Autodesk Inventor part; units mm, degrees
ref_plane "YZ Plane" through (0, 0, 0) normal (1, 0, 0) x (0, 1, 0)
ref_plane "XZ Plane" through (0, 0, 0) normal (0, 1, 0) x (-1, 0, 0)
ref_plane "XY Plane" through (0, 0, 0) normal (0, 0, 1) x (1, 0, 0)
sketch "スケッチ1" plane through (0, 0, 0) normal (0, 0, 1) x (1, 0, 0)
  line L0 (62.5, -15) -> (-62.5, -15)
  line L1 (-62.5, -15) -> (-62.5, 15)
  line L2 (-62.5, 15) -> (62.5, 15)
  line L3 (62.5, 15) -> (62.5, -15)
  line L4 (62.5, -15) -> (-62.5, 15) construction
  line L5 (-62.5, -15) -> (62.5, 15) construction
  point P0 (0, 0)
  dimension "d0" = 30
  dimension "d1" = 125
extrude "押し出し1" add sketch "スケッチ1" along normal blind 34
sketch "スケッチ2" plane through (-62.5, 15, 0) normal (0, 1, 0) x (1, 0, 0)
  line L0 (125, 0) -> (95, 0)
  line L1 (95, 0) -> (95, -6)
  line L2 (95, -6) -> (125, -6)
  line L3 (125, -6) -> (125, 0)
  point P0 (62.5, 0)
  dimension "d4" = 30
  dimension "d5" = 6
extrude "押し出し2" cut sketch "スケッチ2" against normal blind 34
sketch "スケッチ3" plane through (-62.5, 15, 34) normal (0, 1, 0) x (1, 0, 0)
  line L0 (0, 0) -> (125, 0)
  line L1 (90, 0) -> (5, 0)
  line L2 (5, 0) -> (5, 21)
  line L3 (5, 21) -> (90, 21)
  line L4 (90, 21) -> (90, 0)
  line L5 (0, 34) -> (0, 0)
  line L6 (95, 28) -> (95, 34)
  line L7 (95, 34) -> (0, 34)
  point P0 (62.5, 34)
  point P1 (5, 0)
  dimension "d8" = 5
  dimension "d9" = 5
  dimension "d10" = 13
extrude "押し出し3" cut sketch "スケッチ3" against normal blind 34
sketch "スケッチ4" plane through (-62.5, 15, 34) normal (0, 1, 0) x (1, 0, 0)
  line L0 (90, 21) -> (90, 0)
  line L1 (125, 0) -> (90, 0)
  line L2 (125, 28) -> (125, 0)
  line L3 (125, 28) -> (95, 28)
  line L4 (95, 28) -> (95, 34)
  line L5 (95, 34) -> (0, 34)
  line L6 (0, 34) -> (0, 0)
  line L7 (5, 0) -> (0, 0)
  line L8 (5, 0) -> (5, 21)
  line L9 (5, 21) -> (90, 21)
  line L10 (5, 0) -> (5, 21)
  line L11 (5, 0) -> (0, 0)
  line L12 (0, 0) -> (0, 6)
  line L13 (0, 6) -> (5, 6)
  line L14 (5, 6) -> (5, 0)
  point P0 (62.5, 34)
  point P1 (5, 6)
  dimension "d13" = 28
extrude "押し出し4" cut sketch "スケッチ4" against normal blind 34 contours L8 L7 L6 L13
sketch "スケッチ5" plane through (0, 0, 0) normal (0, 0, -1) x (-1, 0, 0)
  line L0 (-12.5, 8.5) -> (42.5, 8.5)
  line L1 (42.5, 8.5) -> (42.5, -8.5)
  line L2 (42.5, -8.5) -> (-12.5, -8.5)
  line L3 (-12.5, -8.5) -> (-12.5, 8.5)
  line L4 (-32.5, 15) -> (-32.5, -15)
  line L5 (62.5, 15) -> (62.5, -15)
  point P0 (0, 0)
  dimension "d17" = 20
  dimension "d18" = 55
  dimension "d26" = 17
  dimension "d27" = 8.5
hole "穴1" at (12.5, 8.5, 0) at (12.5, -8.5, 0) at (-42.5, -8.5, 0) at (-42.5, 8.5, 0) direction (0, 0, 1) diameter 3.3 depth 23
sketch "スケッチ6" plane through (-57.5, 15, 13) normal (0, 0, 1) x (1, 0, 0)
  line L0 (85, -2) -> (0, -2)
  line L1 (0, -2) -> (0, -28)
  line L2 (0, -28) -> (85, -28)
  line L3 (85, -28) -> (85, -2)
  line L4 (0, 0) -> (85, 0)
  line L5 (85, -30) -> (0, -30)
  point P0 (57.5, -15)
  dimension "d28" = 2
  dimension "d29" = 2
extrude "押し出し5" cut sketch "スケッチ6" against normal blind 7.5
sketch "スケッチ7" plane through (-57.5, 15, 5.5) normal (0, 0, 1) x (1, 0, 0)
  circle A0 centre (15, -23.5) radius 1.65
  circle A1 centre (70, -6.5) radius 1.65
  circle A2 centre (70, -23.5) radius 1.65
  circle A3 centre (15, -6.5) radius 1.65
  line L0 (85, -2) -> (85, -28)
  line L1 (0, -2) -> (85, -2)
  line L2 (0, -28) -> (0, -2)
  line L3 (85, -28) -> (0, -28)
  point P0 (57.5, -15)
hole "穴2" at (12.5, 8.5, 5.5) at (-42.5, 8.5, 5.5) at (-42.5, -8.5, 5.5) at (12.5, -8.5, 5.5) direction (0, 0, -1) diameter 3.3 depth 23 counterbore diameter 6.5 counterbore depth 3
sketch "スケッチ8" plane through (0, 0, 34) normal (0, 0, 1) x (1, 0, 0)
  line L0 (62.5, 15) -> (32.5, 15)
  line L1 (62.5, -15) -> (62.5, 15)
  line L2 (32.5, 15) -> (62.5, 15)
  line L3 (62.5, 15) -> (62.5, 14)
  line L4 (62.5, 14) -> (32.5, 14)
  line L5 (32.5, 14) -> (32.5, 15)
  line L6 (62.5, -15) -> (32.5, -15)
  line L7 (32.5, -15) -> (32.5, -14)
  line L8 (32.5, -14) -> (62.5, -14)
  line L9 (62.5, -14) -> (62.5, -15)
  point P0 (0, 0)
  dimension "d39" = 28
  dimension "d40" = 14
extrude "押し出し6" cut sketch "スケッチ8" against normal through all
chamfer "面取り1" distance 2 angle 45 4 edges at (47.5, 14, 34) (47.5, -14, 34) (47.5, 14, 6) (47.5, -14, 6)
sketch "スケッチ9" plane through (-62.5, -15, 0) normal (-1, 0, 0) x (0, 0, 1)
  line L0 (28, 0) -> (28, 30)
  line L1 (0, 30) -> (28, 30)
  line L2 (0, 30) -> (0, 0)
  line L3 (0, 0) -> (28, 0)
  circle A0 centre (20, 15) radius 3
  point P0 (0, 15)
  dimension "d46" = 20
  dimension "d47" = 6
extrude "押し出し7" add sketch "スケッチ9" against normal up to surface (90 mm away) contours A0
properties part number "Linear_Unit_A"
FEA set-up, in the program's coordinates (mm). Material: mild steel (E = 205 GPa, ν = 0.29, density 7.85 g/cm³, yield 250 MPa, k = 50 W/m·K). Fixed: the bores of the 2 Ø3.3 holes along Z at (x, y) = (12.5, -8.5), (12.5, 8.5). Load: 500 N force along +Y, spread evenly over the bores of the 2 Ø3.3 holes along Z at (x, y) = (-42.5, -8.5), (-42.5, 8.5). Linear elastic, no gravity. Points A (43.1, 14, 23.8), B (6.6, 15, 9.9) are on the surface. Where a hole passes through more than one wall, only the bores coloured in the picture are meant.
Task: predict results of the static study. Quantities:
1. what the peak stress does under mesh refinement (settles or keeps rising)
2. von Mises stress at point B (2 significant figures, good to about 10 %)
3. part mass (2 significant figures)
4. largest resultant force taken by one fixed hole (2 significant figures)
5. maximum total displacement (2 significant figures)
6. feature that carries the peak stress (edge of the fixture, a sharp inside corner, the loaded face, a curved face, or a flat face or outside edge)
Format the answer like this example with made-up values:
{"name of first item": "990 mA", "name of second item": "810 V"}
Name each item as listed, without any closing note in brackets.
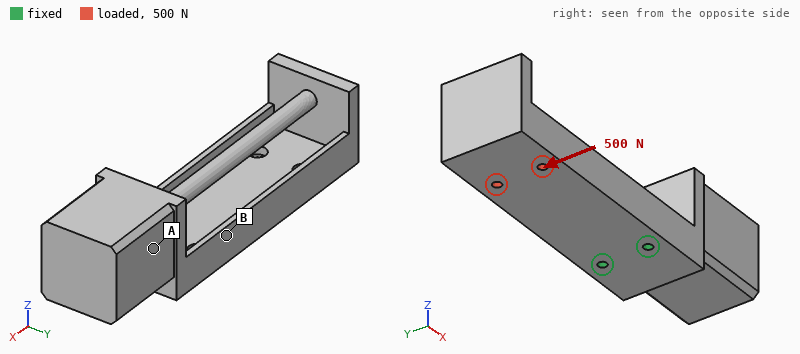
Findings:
{"what the peak stress does under mesh refinement": "keeps rising", "von Mises stress at point B": "13 MPa", "part mass": "400 g", "largest resultant force taken by one fixed hole": "1.5 kN", "maximum total displacement": "26 µm", "feature that carries the peak stress": "edge of the fixture"}
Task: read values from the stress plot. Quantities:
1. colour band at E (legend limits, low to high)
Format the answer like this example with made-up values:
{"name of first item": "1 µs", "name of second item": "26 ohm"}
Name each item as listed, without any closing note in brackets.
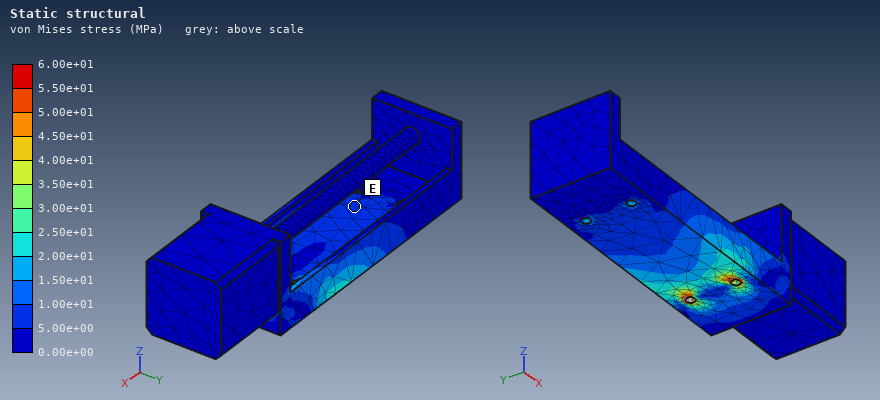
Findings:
{"colour band at E": "5.00e+00 to 1.00e+01 MPa"}
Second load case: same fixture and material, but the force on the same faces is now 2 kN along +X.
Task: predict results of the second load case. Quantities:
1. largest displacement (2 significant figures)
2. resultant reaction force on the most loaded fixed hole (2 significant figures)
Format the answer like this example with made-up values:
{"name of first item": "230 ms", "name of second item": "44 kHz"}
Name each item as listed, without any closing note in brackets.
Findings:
{"largest displacement": "23 µm", "resultant reaction force on the most loaded fixed hole": "1.0 kN"}
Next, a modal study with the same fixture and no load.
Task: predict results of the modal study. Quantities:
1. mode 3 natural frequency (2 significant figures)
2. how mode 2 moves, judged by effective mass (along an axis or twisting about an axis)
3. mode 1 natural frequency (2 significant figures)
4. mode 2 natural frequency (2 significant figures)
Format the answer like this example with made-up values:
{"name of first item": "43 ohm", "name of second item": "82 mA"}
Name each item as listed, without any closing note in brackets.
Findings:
{"mode 3 natural frequency": "1700 Hz", "how mode 2 moves, judged by effective mass": "along Z", "mode 1 natural frequency": "470 Hz", "mode 2 natural frequency": "1700 Hz"}
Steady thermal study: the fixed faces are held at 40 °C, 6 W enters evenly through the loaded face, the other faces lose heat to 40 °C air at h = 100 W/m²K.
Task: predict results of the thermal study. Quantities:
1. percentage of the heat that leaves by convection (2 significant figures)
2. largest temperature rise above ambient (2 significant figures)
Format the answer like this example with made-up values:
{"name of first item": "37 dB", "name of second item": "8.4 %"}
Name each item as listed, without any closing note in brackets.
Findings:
{"percentage of the heat that leaves by convection": "86 %", "largest temperature rise above ambient": "14 K"}
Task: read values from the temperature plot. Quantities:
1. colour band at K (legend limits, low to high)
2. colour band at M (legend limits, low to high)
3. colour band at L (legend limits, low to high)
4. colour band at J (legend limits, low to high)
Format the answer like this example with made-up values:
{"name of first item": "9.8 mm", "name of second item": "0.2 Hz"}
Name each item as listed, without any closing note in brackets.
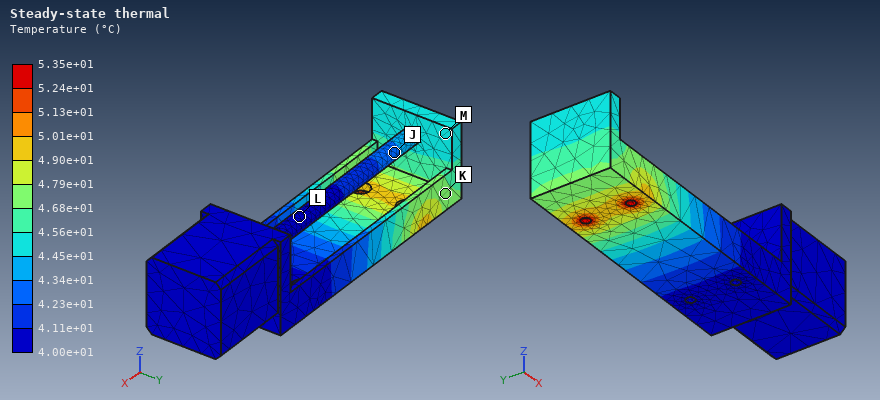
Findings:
{"colour band at K": "4.68e+01 to 4.79e+01 °C", "colour band at M": "4.45e+01 to 4.56e+01 °C", "colour band at L": "4.00e+01 to 4.11e+01 °C", "colour band at J": "4.23e+01 to 4.34e+01 °C"}
